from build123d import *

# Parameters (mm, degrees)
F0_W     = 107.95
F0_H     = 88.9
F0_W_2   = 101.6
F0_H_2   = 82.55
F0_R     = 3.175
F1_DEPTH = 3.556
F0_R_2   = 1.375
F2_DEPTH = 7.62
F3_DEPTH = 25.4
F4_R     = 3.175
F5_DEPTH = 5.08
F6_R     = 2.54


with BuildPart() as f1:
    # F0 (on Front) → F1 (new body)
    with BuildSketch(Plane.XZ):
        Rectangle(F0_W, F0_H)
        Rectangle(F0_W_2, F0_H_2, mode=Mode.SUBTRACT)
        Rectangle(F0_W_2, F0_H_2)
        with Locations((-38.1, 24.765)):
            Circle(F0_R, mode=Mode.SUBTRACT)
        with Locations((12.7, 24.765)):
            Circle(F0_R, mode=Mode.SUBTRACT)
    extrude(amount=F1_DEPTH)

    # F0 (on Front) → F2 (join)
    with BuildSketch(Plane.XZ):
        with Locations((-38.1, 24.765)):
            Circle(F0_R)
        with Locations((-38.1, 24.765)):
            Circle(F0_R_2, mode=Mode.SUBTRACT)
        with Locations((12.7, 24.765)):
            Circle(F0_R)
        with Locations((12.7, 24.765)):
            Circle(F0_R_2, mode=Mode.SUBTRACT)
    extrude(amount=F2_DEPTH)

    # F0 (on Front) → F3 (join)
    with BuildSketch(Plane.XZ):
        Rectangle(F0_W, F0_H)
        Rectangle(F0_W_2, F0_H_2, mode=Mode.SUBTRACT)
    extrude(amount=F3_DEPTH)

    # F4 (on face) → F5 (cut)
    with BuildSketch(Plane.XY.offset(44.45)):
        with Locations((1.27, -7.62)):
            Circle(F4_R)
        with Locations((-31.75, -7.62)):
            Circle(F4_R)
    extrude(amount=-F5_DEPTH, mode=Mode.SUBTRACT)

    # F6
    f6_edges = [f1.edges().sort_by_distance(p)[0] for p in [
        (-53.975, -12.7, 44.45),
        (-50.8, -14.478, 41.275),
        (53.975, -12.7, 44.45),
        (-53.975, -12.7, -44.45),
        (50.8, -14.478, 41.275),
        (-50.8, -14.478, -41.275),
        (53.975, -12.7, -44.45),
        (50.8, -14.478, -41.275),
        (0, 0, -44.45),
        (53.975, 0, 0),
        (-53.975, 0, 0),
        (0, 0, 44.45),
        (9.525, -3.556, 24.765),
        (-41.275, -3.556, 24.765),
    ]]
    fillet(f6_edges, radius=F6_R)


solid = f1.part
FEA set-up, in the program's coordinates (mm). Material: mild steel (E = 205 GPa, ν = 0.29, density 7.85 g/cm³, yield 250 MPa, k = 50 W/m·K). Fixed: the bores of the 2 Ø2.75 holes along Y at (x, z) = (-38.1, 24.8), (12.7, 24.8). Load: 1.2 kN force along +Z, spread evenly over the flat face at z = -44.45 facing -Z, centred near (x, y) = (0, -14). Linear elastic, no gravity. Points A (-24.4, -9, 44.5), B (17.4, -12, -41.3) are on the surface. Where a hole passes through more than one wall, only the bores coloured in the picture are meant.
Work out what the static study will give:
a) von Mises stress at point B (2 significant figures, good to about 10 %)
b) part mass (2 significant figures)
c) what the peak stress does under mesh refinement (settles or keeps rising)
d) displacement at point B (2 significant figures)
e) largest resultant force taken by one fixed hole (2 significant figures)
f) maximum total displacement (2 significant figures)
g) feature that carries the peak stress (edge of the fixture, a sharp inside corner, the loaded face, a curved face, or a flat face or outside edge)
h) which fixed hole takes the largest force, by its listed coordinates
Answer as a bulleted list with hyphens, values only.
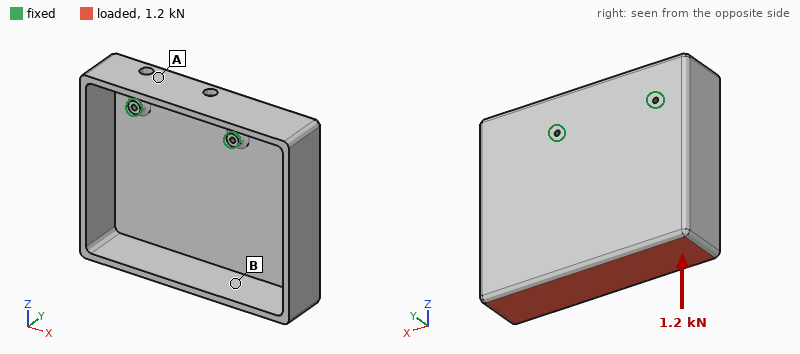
- 19 MPa
- 470 g
- keeps rising
- 0.15 mm
- 900 N
- 0.20 mm
- edge of the fixture
- (12.7, 24.8)
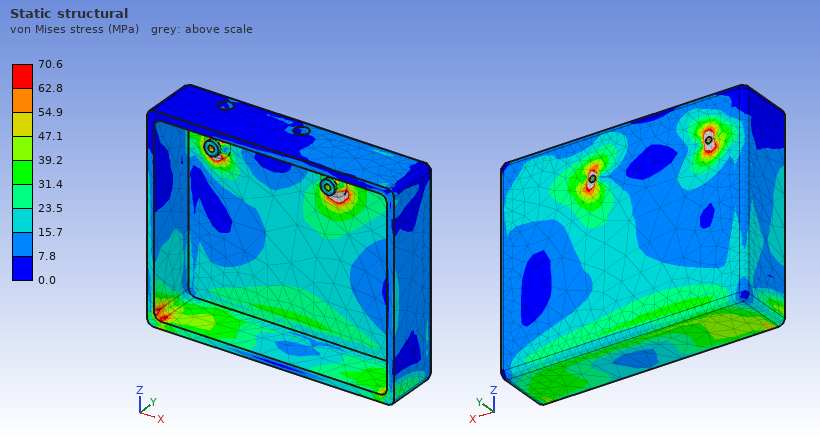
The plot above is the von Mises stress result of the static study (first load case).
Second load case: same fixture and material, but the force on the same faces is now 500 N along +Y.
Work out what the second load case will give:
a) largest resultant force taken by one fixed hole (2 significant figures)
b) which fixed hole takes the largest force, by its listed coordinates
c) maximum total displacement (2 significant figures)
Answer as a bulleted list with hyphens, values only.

- 370 N
- (12.7, 24.8)
- 0.45 mm
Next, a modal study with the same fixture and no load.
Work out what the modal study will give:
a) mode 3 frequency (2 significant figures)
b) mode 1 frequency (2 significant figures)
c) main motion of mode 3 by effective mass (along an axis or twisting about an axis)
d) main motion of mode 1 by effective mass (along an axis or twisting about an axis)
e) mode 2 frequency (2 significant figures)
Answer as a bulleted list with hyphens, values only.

- 1900 Hz
- 480 Hz
- along Y
- along Y
- 850 Hz
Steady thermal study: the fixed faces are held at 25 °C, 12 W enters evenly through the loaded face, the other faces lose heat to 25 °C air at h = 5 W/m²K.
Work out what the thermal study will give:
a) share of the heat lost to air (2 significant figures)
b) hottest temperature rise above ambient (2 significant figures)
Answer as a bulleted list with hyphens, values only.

- 26 %
- 43 K
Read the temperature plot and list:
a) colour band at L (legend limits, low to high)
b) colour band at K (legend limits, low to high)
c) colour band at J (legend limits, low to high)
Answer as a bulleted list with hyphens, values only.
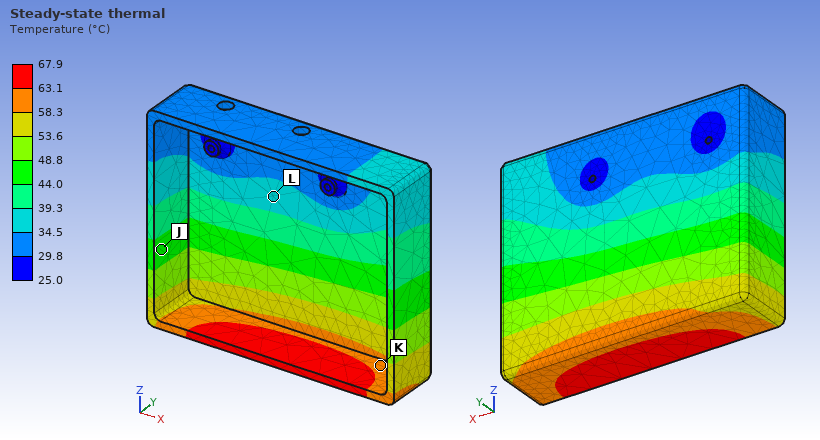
- 34.5 to 39.3 °C
- 58.3 to 63.1 °C
- 44.0 to 48.8 °C
